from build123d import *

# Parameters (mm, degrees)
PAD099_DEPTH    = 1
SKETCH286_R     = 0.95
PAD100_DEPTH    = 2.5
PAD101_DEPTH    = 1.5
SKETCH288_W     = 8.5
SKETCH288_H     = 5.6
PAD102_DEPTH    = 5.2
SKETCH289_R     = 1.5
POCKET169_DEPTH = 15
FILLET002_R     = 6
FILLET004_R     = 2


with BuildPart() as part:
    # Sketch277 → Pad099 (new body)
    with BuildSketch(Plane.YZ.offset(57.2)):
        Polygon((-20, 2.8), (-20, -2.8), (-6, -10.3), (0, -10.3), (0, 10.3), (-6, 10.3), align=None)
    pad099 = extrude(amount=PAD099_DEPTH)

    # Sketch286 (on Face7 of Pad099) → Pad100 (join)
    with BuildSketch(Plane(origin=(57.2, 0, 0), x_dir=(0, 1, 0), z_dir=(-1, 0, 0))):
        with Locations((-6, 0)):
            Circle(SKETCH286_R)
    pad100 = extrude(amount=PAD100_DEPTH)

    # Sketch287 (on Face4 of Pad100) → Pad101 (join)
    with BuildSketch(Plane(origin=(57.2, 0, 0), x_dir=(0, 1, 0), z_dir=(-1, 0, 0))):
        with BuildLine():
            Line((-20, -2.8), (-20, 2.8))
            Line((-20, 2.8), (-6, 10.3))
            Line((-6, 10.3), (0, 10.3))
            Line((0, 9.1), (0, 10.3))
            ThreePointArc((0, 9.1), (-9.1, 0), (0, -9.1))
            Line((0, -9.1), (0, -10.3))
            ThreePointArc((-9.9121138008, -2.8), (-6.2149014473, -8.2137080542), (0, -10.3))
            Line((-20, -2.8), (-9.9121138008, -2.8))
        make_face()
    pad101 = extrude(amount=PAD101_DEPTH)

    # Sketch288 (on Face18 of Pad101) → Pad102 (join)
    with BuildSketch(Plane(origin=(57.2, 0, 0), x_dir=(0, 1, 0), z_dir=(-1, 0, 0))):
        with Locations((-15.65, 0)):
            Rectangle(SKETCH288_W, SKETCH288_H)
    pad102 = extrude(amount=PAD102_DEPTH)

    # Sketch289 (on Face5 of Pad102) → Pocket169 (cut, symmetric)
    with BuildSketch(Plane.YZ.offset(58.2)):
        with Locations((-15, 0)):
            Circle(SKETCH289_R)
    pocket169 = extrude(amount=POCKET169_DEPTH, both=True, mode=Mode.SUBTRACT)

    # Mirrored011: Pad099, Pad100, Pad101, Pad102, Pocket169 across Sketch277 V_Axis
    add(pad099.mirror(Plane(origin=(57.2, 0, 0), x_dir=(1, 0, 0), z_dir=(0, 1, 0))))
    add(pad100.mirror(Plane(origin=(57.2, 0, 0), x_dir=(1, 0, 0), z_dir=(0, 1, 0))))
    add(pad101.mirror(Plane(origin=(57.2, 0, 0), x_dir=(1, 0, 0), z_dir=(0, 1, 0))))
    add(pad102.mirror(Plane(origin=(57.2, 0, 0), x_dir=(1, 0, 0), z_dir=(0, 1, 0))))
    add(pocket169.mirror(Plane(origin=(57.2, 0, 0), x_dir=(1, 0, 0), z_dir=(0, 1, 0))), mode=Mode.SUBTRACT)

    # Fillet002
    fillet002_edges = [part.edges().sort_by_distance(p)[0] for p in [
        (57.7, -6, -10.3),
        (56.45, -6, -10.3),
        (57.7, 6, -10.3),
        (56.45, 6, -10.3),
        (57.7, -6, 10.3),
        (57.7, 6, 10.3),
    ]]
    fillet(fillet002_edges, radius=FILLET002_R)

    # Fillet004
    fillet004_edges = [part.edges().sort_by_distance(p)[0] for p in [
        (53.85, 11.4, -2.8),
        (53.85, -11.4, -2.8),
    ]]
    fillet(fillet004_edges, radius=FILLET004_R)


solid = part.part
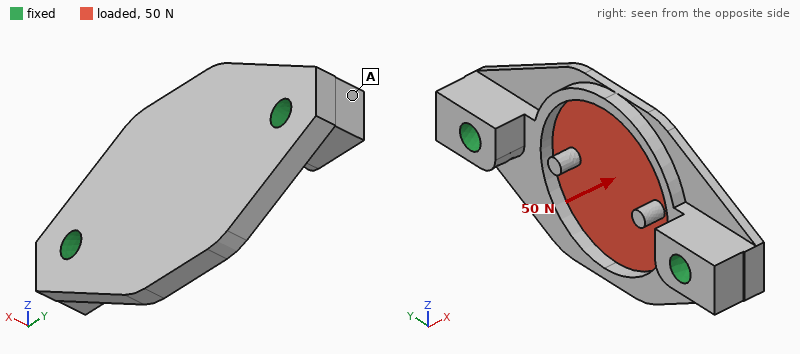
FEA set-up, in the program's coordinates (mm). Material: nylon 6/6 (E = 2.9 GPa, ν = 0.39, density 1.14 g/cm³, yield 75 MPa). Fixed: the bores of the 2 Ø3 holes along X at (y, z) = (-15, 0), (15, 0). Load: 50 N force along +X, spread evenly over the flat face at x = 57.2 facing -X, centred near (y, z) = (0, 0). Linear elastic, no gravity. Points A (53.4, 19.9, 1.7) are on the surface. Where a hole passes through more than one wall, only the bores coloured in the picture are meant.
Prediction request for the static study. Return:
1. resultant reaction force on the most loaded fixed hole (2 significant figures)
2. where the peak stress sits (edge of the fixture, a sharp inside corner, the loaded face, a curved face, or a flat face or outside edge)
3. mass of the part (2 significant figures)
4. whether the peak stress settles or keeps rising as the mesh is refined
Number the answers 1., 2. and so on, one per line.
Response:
1. 32 N
2. a sharp inside corner
3. 1.5 g
4. keeps rising
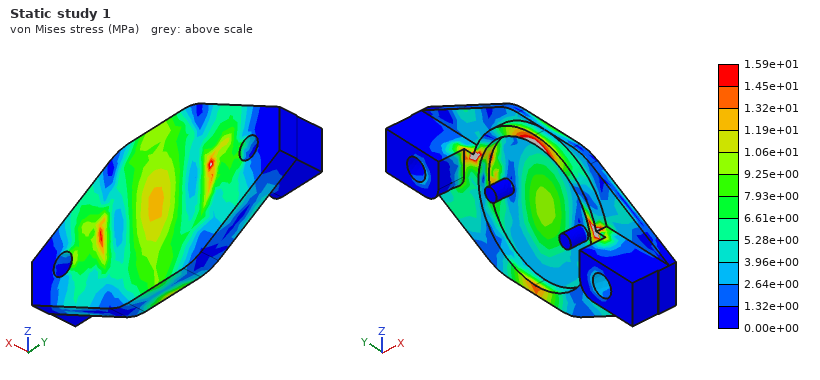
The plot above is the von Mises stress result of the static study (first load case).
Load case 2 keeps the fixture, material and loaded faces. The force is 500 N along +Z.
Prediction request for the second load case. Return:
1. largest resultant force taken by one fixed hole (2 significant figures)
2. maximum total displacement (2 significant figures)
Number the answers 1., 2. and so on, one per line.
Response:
1. 250 N
2. 0.18 mm
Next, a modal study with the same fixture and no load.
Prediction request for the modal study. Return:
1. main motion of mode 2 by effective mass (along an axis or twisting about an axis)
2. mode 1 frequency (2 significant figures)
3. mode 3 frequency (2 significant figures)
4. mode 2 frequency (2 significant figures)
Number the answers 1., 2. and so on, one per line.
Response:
1. along X
2. 3500 Hz
3. 7600 Hz
4. 4300 Hz
